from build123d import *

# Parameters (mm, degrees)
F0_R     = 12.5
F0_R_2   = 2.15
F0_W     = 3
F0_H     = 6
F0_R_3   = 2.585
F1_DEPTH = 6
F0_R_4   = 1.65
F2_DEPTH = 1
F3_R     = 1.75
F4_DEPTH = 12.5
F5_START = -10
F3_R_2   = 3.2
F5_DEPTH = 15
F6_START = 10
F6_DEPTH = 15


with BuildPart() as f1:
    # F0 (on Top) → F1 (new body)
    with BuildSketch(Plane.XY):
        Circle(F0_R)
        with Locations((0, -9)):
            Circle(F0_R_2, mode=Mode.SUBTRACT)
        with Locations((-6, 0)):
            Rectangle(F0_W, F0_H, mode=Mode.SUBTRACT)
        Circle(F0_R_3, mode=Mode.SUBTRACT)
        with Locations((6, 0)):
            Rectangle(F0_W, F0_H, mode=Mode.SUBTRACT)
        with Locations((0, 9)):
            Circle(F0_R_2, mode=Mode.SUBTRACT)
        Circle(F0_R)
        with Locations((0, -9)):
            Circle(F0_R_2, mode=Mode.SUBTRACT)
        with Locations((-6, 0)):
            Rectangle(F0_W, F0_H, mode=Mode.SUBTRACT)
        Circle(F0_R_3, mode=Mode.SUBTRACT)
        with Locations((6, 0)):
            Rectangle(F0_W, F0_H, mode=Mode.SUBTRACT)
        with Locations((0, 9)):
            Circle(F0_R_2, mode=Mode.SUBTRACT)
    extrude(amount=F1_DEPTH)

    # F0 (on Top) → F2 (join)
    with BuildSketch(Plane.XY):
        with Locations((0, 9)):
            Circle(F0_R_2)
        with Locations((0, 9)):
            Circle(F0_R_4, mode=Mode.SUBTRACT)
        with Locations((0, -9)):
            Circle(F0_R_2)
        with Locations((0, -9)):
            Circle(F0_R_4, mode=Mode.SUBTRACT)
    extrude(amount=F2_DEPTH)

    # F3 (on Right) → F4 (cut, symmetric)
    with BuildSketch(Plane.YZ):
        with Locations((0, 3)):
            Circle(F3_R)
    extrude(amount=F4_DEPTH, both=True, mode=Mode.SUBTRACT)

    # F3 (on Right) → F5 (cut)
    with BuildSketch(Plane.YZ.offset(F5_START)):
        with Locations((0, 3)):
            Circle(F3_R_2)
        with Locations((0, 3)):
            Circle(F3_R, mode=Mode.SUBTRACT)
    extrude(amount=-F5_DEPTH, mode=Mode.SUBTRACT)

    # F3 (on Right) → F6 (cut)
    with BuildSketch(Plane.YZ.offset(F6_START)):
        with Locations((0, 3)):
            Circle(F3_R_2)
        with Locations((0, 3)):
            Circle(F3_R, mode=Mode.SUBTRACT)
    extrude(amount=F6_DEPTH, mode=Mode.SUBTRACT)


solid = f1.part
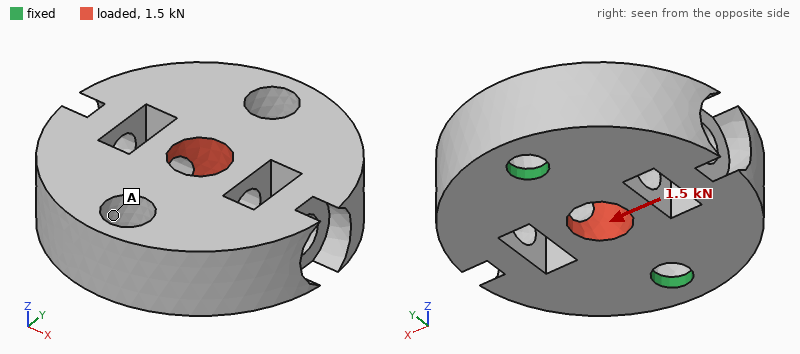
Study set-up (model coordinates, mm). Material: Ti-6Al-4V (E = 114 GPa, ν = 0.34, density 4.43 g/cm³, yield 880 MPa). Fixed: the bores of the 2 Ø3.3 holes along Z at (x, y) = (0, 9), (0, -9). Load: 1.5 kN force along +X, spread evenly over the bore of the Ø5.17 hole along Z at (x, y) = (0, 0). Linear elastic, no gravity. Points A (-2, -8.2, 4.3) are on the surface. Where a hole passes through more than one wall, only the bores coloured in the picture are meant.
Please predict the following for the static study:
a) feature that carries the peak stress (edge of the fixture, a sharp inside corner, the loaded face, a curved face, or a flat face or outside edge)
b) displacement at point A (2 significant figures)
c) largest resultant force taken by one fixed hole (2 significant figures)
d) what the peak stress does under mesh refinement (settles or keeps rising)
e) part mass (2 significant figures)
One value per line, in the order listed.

edge of the fixture
13 µm
750 N
keeps rising
9.8 g
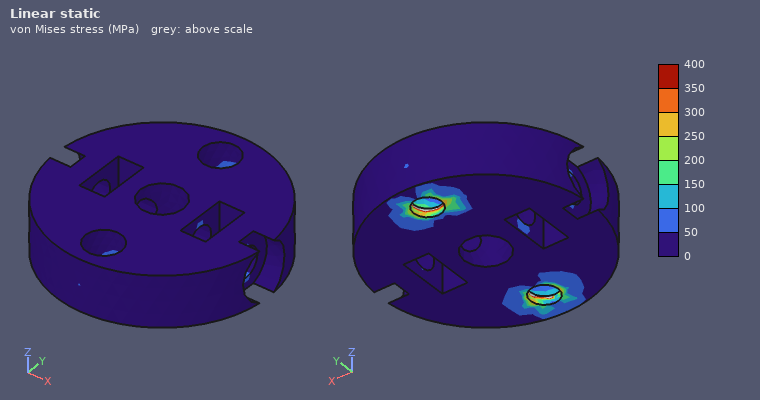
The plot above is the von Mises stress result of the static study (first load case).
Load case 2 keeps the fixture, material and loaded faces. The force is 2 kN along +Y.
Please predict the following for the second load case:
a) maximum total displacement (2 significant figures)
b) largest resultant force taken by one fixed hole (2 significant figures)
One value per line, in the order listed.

5.8 µm
1.0 kN
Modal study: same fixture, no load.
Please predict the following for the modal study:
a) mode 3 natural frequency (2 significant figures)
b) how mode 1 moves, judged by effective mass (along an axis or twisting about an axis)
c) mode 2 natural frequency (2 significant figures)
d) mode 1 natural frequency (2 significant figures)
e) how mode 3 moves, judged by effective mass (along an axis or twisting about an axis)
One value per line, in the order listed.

27 kHz
along X
25 kHz
8900 Hz
along Z
